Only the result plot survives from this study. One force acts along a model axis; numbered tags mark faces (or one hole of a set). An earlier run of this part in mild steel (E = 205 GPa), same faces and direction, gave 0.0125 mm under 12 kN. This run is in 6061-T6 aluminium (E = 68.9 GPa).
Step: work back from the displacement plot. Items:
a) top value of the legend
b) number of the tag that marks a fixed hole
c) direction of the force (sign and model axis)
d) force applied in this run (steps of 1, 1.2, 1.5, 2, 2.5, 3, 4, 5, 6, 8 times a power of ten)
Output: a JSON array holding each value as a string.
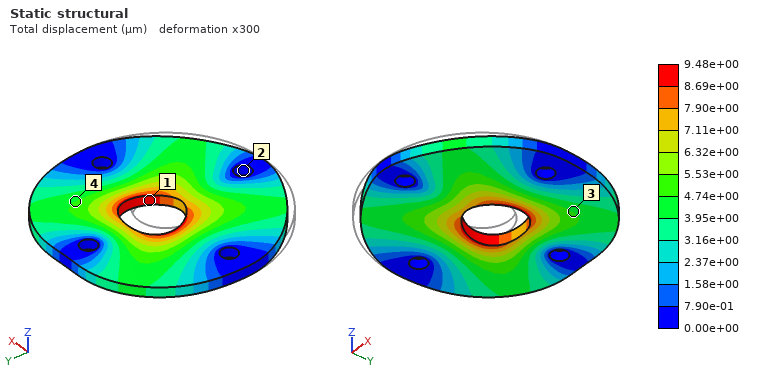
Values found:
["9.48e+00 µm", "2", "+Y", "3 kN"]
